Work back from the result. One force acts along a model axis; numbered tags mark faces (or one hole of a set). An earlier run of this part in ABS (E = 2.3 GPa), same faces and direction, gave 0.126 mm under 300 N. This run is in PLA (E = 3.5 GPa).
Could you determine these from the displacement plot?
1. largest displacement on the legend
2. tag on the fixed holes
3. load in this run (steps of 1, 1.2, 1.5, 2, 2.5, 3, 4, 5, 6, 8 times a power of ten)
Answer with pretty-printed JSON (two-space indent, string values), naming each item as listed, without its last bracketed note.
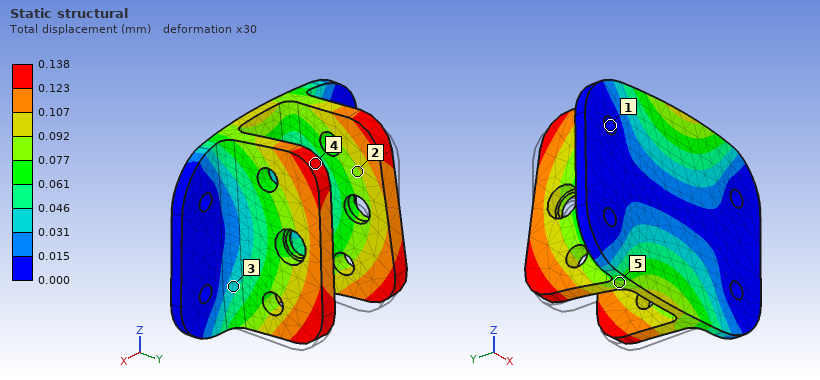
{
  "largest displacement on the legend": "0.138 mm",
  "tag on the fixed holes": "1",
  "load in this run": "500 N"
}
